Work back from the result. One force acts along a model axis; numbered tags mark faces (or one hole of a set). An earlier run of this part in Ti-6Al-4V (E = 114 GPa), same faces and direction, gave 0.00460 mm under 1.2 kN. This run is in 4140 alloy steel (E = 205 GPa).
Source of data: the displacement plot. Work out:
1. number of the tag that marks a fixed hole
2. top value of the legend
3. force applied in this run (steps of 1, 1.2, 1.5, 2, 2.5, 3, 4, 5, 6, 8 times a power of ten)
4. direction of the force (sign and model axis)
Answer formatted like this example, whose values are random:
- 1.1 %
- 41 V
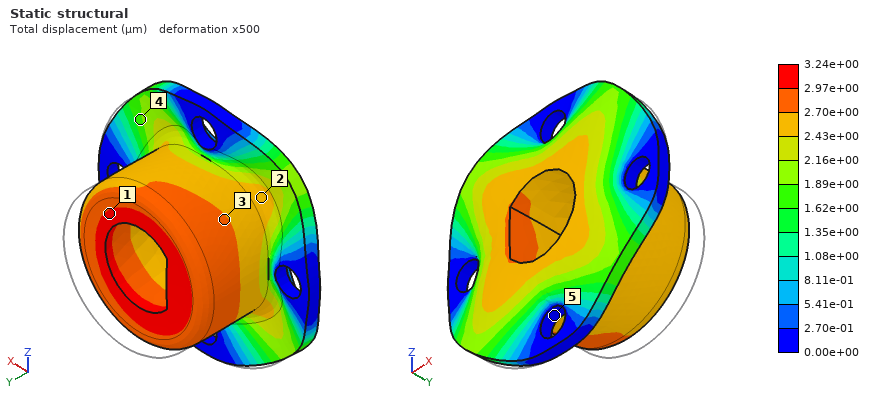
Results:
- 5
- 3.24e+00 µm
- 1.5 kN
- -Y
